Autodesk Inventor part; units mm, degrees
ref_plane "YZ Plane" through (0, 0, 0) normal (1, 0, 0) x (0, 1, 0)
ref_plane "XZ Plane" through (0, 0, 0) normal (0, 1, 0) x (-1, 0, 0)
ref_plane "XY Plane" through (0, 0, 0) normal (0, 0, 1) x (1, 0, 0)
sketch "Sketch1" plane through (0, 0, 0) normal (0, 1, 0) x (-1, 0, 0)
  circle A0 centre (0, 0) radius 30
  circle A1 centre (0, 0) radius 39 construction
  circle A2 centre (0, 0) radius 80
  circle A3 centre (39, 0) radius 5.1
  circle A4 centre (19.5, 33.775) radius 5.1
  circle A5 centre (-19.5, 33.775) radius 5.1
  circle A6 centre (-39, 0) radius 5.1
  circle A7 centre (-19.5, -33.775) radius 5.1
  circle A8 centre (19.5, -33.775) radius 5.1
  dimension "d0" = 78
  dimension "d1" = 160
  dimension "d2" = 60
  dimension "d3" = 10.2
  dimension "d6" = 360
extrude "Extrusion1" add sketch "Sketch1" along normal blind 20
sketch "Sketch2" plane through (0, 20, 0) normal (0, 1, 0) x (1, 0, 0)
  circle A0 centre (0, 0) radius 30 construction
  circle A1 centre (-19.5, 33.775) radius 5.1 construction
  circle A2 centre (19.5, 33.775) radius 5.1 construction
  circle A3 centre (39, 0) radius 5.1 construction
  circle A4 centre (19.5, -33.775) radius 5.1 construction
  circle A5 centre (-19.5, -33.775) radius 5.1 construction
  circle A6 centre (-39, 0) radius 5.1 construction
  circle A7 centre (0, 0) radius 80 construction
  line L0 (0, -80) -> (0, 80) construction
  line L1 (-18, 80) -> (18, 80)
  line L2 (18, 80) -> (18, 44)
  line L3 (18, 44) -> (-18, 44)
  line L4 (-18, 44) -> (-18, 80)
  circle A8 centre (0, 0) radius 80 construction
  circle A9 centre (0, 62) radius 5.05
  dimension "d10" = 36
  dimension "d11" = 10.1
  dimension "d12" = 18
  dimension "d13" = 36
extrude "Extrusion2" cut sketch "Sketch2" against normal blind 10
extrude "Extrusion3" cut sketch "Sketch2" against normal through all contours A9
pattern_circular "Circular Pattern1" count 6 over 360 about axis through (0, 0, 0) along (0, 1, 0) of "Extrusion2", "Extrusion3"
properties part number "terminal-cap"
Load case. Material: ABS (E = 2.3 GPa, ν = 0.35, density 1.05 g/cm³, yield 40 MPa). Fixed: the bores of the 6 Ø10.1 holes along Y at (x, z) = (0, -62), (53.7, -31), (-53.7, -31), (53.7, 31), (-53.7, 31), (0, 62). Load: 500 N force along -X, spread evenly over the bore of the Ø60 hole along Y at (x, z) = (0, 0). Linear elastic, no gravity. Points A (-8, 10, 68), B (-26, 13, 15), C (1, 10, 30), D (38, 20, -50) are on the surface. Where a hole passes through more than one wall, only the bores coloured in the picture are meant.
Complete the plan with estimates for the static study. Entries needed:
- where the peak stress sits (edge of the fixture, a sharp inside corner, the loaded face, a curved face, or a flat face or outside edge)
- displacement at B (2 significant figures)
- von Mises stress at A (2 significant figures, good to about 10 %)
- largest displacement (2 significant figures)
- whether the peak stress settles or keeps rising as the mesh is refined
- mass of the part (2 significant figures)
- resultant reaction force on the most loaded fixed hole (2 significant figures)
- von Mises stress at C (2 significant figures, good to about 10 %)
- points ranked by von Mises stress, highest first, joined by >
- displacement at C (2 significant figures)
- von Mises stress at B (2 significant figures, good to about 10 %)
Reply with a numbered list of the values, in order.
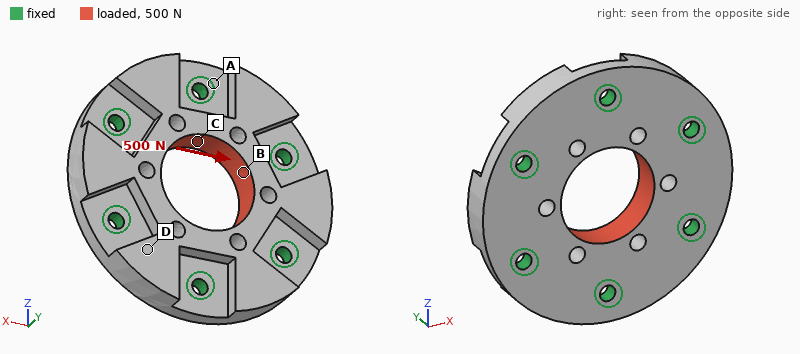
1. edge of the fixture
2. 7.0 µm
3. 0.13 MPa
4. 10 µm
5. keeps rising
6. 270 g
7. 100 N
8. 0.29 MPa
9. C > B > A > D
10. 5.4 µm
11. 0.21 MPa
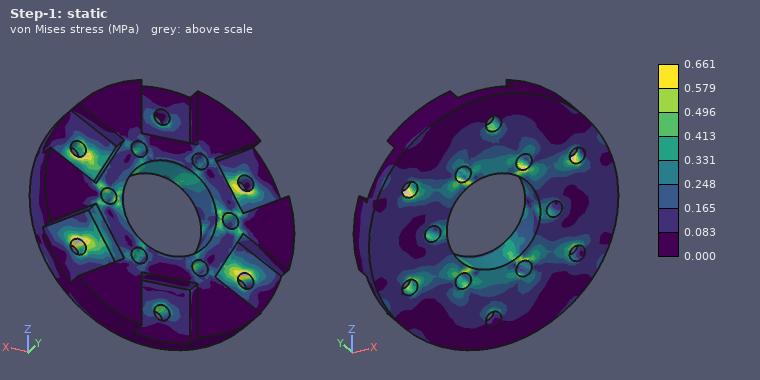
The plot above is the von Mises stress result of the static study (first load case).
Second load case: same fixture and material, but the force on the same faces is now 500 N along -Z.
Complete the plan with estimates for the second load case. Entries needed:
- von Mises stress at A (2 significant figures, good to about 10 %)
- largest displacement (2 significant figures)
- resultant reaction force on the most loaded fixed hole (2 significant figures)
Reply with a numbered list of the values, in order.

1. 0.28 MPa
2. 9.1 µm
3. 110 N
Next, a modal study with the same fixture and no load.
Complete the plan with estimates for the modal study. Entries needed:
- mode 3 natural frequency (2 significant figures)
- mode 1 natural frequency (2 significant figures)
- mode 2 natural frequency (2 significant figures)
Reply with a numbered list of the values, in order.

1. 2500 Hz
2. 2300 Hz
3. 2500 Hz
